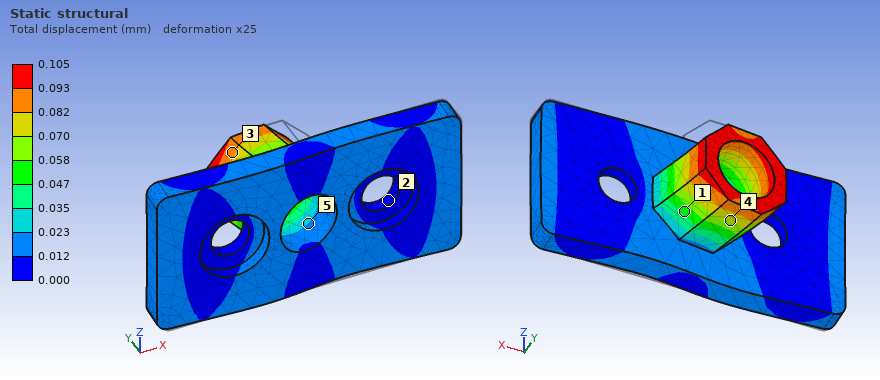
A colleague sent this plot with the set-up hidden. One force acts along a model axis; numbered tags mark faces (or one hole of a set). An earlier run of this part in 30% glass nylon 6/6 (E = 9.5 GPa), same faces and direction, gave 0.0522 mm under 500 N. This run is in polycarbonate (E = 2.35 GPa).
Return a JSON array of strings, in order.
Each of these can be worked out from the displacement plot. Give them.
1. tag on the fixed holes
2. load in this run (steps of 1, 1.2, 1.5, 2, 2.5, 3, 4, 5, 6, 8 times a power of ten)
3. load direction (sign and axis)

["2", "250 N", "-X"]
